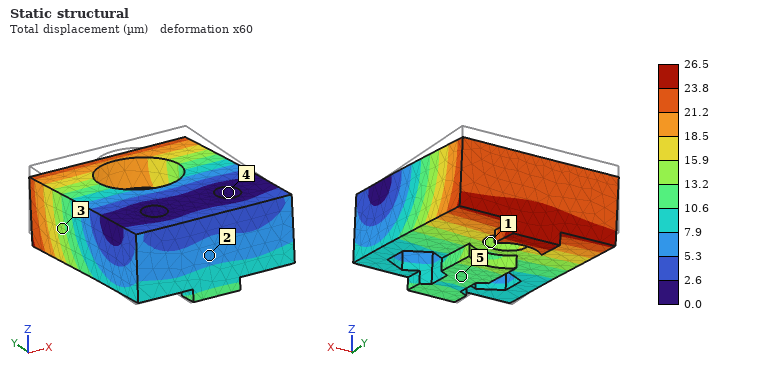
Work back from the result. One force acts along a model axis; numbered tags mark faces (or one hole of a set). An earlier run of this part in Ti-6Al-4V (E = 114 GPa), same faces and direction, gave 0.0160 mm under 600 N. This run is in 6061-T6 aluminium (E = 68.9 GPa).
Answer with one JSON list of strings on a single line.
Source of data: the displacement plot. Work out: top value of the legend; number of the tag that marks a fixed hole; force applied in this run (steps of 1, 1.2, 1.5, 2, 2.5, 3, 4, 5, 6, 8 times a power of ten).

["26.5 µm", "4", "600 N"]
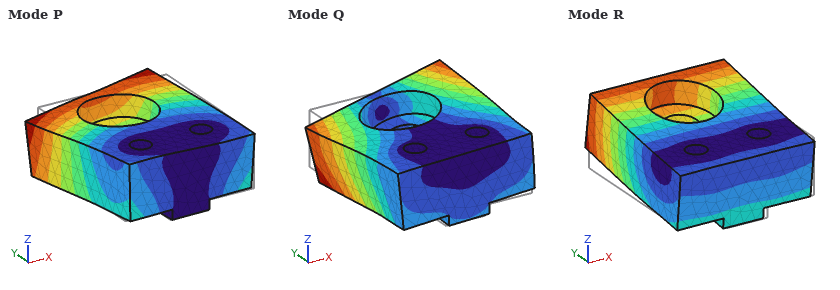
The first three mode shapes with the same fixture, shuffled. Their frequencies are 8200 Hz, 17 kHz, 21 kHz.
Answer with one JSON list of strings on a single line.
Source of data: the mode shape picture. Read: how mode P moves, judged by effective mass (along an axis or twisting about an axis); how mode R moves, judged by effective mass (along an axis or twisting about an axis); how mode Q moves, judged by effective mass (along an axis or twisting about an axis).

["along X", "along Z", "along X"]
